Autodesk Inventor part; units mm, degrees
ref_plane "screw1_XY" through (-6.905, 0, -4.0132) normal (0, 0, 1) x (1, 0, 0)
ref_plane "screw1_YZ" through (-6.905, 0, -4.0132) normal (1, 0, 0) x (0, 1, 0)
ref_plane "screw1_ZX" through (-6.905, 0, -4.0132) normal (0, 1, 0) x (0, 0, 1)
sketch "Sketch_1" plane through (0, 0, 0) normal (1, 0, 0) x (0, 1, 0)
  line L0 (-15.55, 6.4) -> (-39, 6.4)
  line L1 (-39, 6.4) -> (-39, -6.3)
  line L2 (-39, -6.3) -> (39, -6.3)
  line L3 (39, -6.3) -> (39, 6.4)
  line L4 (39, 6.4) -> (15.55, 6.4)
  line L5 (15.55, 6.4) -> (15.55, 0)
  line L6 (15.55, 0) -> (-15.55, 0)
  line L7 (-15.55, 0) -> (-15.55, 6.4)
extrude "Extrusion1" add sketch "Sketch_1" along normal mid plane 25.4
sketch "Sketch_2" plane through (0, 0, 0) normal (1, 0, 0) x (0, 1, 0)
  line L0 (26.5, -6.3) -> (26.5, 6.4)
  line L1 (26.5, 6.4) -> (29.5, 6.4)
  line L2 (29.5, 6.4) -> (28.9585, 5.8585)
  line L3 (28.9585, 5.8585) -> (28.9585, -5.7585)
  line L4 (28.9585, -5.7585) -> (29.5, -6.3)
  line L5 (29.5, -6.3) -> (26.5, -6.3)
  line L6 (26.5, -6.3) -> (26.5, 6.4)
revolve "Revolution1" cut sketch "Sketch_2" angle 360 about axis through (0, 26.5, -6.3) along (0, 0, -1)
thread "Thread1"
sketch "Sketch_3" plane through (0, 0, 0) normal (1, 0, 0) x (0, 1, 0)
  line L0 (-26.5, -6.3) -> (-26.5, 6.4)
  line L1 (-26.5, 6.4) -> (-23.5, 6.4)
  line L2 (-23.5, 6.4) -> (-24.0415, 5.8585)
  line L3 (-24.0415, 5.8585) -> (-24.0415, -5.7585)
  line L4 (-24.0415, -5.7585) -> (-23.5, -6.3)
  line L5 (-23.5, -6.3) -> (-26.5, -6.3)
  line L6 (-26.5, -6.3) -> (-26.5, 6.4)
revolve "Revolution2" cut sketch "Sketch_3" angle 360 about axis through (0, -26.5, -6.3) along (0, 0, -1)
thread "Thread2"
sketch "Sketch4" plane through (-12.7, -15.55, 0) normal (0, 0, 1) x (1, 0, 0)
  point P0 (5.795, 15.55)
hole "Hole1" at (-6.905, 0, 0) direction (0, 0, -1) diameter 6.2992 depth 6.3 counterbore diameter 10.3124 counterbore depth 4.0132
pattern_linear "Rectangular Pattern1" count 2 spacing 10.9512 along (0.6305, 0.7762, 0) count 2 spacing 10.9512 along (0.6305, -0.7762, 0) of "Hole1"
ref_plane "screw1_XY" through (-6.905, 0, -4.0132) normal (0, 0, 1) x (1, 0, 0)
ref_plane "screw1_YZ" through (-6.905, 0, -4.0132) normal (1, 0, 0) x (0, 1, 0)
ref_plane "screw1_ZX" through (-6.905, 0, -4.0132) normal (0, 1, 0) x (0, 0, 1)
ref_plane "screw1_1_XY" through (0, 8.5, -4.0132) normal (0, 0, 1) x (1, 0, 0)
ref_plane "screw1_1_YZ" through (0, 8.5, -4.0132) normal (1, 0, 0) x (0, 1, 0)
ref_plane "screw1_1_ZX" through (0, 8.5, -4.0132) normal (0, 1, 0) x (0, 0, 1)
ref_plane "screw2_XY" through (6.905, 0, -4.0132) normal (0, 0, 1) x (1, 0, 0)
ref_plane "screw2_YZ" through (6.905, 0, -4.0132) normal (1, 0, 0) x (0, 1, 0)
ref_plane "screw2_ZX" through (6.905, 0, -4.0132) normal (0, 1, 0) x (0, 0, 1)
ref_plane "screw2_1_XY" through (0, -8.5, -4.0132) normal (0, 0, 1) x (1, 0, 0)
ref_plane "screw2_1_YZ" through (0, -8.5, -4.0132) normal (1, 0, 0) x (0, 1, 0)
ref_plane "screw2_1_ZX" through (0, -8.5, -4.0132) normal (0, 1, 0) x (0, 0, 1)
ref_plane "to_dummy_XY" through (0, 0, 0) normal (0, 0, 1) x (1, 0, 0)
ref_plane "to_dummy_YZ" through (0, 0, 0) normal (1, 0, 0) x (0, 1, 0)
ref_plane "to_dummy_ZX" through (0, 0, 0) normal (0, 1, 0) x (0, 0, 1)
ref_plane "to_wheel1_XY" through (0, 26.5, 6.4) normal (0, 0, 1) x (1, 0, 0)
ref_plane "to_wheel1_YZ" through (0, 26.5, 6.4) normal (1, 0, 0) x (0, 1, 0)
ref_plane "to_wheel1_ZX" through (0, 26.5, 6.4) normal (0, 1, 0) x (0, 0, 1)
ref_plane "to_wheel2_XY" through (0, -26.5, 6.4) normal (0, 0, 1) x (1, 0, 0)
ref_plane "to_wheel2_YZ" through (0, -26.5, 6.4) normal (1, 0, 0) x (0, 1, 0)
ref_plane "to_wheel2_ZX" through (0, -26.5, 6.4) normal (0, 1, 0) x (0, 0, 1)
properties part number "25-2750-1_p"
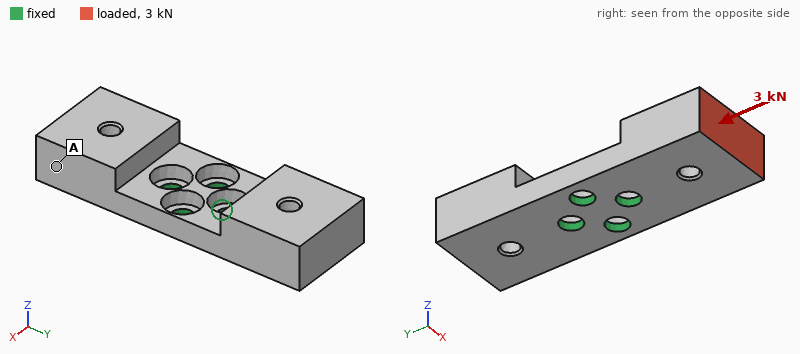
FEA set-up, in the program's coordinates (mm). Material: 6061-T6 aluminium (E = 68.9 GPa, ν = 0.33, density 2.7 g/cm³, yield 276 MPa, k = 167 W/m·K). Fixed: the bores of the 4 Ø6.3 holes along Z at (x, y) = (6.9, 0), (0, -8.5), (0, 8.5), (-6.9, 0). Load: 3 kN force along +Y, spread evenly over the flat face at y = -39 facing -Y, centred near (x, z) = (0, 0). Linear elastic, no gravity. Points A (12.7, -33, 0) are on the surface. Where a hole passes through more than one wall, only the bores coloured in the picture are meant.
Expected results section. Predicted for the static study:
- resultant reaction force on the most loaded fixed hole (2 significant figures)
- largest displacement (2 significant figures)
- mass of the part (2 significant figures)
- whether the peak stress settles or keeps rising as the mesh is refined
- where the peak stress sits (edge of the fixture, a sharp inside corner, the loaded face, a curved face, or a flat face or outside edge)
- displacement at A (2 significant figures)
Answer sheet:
1.4 kN
0.17 mm
49 g
keeps rising
edge of the fixture
0.12 mm
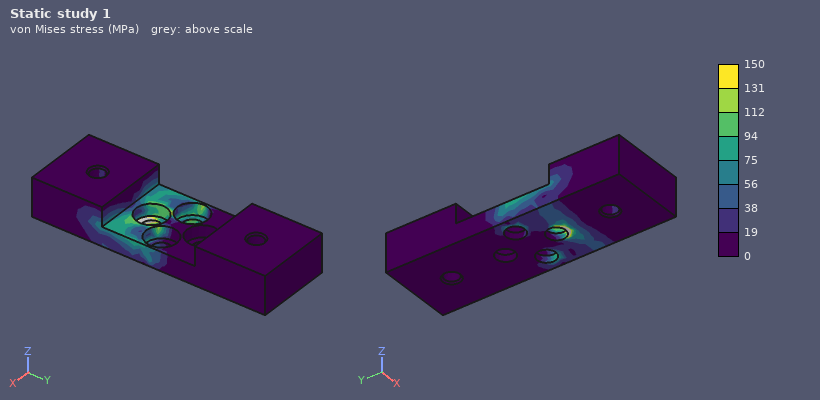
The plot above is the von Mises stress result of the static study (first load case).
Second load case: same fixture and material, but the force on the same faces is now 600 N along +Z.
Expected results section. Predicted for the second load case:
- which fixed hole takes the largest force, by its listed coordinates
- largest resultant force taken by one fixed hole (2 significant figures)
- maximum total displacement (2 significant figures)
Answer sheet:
(0, -8.5)
2.4 kN
0.22 mm
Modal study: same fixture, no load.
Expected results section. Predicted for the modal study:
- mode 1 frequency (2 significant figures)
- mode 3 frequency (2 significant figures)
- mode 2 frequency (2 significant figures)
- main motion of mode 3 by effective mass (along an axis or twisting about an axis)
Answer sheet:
2900 Hz
6900 Hz
2900 Hz
twisting about Z
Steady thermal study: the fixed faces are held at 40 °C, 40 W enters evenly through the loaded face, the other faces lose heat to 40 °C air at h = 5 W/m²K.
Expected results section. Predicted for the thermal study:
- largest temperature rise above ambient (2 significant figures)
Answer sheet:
39 K
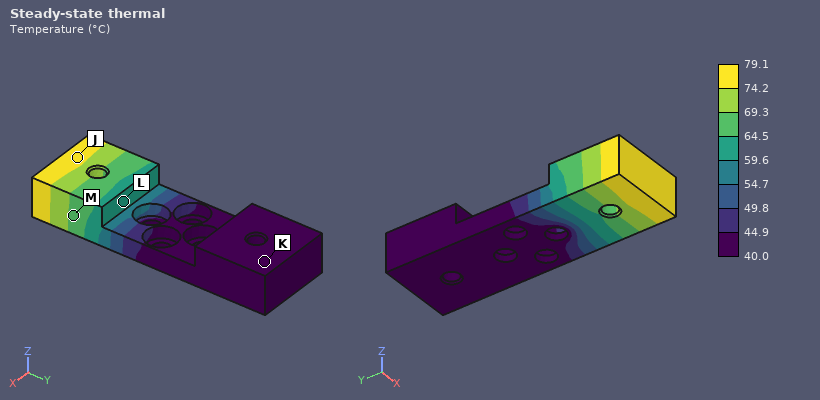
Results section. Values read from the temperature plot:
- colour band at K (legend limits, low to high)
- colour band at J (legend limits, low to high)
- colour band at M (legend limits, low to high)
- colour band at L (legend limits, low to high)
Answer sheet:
40.0 to 44.9 °C
74.2 to 79.1 °C
64.5 to 69.3 °C
59.6 to 64.5 °C
